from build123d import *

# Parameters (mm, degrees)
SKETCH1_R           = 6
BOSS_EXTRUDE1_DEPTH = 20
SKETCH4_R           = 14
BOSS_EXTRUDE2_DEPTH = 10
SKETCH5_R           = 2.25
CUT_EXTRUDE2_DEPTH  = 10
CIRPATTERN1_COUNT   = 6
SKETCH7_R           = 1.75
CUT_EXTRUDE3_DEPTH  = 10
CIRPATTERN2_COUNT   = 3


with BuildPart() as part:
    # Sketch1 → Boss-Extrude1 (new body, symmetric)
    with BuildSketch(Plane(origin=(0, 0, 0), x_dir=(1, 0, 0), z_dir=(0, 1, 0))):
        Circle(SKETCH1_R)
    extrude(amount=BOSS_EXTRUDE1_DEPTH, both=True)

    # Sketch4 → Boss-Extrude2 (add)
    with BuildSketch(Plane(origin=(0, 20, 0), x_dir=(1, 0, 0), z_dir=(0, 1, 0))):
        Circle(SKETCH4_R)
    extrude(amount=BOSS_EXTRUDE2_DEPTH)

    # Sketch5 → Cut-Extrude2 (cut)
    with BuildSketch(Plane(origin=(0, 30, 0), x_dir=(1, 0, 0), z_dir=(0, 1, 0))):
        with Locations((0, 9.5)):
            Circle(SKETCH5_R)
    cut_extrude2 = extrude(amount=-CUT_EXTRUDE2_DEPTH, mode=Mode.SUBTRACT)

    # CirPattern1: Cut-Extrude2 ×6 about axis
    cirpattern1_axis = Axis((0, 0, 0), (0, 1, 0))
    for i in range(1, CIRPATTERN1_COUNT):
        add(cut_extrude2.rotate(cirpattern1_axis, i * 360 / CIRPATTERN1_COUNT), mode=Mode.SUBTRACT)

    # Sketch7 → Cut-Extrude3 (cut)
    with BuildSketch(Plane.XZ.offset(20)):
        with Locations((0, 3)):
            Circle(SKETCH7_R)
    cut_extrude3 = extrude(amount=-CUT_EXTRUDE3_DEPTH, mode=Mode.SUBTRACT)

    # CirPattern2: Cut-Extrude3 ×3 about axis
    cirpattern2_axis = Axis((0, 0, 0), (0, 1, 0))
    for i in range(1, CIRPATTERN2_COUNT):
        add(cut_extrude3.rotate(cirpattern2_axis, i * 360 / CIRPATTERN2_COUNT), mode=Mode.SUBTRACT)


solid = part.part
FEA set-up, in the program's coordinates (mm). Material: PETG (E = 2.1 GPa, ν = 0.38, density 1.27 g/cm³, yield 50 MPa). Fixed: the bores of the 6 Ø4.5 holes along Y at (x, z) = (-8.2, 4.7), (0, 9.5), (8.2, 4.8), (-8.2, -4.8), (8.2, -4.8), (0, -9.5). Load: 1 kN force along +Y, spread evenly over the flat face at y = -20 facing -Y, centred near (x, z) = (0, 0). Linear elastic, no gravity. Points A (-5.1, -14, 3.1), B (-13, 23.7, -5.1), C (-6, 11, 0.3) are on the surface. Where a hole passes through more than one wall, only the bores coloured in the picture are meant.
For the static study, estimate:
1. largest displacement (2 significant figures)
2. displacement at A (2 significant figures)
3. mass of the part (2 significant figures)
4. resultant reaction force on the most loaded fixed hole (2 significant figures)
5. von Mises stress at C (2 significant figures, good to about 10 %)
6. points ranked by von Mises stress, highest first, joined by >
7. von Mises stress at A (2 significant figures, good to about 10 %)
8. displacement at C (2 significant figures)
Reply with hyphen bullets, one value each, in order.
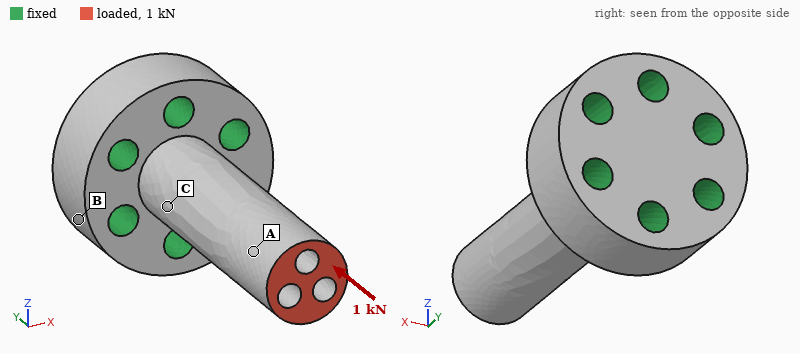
- 0.20 mm
- 0.17 mm
- 12 g
- 210 N
- 8.7 MPa
- A > C > B
- 11 MPa
- 0.054 mm
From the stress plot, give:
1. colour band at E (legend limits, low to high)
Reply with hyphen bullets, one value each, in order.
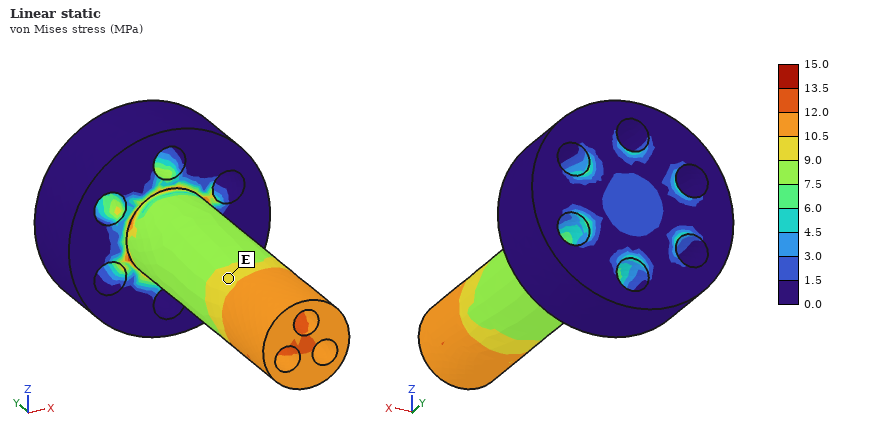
- 9.0 to 10.5 MPa
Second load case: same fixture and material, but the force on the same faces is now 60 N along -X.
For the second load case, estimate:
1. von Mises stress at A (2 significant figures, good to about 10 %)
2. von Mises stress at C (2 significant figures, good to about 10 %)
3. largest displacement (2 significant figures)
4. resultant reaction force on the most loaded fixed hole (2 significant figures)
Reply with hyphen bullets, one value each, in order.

- 2.3 MPa
- 11 MPa
- 0.75 mm
- 97 N
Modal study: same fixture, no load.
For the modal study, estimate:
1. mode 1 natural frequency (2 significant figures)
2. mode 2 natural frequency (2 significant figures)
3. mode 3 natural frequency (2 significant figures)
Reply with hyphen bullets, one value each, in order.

- 1300 Hz
- 1300 Hz
- 4800 Hz
